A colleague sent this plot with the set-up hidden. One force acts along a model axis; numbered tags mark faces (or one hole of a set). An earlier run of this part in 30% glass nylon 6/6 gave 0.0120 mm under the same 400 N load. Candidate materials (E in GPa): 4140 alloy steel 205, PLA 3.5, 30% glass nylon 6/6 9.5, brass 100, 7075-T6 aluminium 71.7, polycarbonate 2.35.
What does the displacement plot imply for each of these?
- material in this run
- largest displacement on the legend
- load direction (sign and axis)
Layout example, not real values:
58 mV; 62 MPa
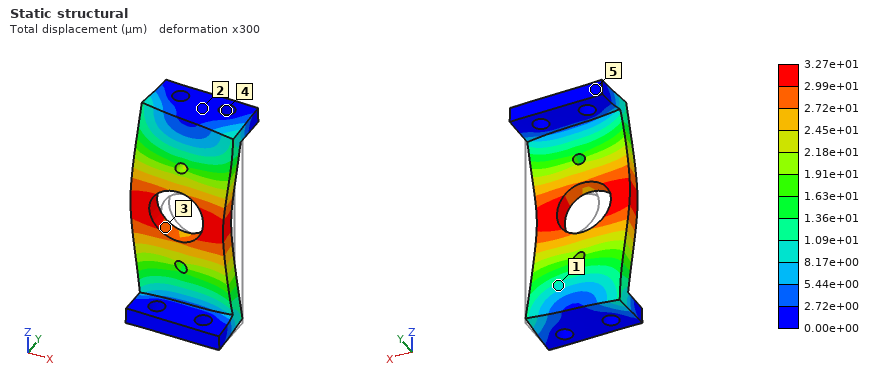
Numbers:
PLA; 3.27e+01 µm; -X
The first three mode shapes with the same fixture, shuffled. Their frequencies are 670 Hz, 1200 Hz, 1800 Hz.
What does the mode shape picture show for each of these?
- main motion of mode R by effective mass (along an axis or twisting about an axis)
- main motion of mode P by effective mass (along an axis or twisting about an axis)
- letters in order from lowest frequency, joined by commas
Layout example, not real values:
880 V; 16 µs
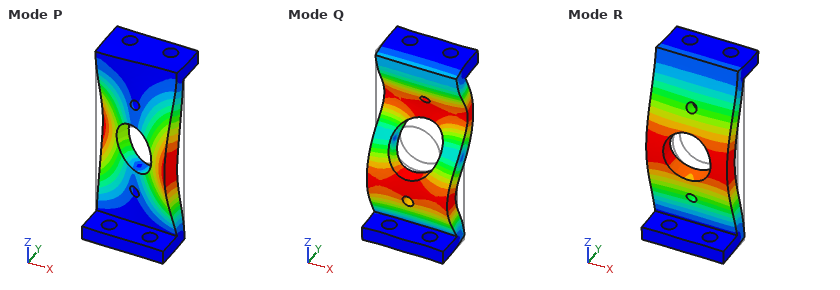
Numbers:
along Y; twisting about Z; R, P, Q
